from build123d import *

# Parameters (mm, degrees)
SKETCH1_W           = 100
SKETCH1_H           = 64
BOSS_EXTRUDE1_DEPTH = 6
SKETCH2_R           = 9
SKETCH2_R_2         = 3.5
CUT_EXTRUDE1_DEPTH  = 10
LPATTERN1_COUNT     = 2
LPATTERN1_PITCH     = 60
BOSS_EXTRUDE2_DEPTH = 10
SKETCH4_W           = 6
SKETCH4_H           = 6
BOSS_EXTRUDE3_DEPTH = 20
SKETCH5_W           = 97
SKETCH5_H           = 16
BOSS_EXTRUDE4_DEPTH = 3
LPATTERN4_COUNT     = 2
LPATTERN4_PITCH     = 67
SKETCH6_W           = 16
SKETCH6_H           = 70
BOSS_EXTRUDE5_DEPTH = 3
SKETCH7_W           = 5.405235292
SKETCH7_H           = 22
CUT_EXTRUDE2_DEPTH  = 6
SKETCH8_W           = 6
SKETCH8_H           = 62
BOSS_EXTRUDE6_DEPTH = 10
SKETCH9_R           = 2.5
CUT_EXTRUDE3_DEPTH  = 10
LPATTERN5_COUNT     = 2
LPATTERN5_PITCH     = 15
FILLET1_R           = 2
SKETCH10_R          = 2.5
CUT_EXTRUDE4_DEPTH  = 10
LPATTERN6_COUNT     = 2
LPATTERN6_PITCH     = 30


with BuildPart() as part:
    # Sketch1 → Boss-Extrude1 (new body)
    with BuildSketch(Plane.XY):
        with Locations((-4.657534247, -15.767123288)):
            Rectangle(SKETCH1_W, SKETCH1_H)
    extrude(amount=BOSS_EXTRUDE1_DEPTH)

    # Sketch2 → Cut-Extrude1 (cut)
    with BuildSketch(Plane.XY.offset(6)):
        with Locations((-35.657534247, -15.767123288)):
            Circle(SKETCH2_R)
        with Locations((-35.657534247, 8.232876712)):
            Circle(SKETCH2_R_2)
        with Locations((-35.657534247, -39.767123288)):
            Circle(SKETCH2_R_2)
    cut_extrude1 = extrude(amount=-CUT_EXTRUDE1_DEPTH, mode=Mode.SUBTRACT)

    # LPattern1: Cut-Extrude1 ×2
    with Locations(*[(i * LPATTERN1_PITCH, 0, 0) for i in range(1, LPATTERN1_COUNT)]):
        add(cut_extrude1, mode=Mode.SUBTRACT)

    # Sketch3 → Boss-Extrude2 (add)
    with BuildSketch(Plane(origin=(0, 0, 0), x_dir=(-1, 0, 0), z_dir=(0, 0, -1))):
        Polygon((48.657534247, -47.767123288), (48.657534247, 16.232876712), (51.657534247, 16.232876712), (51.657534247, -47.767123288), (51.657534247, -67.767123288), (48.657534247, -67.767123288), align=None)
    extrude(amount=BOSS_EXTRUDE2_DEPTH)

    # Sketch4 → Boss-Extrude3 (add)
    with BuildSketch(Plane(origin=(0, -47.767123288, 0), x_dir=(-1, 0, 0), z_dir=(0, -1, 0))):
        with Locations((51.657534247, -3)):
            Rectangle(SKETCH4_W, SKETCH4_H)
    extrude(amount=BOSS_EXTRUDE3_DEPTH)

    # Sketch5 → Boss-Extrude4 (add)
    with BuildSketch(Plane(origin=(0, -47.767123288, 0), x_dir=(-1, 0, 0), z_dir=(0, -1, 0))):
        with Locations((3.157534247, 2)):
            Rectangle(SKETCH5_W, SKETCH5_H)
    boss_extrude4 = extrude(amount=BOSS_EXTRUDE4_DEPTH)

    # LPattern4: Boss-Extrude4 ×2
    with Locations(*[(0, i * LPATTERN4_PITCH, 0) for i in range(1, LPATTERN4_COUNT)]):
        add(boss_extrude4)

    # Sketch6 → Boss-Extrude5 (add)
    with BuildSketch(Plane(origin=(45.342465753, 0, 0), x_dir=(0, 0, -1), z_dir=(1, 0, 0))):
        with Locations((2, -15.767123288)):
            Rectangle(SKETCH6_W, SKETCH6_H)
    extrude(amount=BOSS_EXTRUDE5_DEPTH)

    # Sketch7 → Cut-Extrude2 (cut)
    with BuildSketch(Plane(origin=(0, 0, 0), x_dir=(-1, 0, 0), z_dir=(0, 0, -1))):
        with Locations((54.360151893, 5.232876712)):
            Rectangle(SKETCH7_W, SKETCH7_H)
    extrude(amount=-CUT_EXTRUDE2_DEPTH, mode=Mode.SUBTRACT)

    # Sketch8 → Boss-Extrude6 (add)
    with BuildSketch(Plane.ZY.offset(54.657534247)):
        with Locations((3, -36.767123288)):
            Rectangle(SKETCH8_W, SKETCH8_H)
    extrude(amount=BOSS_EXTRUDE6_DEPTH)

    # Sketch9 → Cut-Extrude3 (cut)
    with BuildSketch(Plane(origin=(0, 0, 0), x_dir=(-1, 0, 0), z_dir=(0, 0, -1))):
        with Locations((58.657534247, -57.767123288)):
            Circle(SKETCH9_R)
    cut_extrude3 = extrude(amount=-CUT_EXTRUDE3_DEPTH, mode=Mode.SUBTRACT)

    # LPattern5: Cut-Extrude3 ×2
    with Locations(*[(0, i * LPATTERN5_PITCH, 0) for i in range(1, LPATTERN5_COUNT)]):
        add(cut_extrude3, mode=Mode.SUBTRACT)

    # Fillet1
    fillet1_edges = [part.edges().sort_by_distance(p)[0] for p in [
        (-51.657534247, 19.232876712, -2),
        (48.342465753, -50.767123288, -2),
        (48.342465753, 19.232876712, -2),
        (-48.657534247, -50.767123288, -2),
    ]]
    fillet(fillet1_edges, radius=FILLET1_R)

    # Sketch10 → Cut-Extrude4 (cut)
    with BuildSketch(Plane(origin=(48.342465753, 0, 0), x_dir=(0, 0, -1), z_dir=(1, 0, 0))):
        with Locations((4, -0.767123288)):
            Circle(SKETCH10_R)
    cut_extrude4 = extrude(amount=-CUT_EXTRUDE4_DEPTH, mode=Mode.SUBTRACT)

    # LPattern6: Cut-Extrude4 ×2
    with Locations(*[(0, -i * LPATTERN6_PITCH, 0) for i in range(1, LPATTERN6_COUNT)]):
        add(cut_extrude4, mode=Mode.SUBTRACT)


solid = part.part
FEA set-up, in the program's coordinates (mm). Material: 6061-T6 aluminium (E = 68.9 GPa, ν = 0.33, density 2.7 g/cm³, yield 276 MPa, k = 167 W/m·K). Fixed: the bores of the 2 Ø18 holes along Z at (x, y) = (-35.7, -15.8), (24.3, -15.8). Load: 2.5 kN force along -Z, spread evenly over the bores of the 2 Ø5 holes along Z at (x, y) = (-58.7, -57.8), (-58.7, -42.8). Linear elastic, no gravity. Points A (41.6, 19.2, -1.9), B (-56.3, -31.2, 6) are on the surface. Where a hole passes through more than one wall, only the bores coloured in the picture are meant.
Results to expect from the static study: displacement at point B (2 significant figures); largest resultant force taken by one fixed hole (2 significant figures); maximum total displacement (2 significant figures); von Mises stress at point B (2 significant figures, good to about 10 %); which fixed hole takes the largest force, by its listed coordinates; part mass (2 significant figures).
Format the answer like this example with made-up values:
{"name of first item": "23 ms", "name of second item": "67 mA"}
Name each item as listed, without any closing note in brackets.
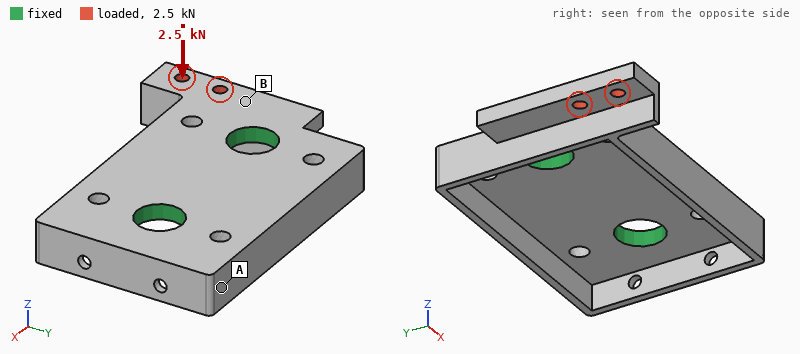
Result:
{"displacement at point B": "0.15 mm", "largest resultant force taken by one fixed hole": "2.9 kN", "maximum total displacement": "0.68 mm", "von Mises stress at point B": "90 MPa", "which fixed hole takes the largest force, by its listed coordinates": "(-35.7, -15.8)", "part mass": "140 g"}
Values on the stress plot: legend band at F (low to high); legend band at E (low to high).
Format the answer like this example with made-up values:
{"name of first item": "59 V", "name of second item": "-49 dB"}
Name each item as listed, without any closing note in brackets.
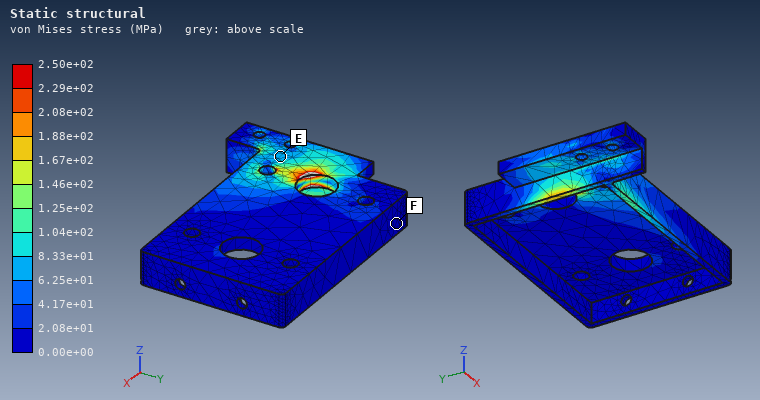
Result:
{"legend band at F": "0.00e+00 to 2.08e+01 MPa", "legend band at E": "6.25e+01 to 8.33e+01 MPa"}
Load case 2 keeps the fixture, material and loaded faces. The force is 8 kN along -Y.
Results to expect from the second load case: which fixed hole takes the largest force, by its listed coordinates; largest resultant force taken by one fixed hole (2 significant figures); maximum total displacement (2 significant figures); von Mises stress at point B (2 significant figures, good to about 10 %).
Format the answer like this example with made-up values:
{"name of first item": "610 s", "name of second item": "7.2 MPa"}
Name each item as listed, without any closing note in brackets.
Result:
{"which fixed hole takes the largest force, by its listed coordinates": "(-35.7, -15.8)", "largest resultant force taken by one fixed hole": "9.6 kN", "maximum total displacement": "0.13 mm", "von Mises stress at point B": "67 MPa"}
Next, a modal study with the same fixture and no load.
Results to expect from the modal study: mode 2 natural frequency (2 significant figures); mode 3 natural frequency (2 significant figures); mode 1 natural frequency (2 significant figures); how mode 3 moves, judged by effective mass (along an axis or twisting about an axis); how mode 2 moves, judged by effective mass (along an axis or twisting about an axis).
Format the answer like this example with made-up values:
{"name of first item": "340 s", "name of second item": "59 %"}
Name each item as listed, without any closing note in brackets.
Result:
{"mode 2 natural frequency": "4300 Hz", "mode 3 natural frequency": "5100 Hz", "mode 1 natural frequency": "3500 Hz", "how mode 3 moves, judged by effective mass": "along Z", "how mode 2 moves, judged by effective mass": "twisting about X"}
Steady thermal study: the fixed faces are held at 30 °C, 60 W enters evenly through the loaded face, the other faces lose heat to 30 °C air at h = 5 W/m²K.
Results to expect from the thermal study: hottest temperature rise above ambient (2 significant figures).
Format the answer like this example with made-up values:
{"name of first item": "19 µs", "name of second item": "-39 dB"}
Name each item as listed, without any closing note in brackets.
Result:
{"hottest temperature rise above ambient": "69 K"}
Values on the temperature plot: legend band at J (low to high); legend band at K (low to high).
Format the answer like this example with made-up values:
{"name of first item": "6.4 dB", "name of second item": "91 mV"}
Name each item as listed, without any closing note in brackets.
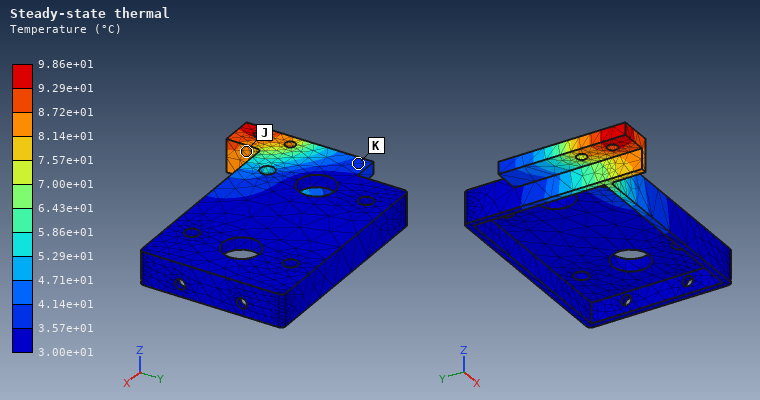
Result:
{"legend band at J": "8.14e+01 to 8.72e+01 °C", "legend band at K": "3.57e+01 to 4.14e+01 °C"}
